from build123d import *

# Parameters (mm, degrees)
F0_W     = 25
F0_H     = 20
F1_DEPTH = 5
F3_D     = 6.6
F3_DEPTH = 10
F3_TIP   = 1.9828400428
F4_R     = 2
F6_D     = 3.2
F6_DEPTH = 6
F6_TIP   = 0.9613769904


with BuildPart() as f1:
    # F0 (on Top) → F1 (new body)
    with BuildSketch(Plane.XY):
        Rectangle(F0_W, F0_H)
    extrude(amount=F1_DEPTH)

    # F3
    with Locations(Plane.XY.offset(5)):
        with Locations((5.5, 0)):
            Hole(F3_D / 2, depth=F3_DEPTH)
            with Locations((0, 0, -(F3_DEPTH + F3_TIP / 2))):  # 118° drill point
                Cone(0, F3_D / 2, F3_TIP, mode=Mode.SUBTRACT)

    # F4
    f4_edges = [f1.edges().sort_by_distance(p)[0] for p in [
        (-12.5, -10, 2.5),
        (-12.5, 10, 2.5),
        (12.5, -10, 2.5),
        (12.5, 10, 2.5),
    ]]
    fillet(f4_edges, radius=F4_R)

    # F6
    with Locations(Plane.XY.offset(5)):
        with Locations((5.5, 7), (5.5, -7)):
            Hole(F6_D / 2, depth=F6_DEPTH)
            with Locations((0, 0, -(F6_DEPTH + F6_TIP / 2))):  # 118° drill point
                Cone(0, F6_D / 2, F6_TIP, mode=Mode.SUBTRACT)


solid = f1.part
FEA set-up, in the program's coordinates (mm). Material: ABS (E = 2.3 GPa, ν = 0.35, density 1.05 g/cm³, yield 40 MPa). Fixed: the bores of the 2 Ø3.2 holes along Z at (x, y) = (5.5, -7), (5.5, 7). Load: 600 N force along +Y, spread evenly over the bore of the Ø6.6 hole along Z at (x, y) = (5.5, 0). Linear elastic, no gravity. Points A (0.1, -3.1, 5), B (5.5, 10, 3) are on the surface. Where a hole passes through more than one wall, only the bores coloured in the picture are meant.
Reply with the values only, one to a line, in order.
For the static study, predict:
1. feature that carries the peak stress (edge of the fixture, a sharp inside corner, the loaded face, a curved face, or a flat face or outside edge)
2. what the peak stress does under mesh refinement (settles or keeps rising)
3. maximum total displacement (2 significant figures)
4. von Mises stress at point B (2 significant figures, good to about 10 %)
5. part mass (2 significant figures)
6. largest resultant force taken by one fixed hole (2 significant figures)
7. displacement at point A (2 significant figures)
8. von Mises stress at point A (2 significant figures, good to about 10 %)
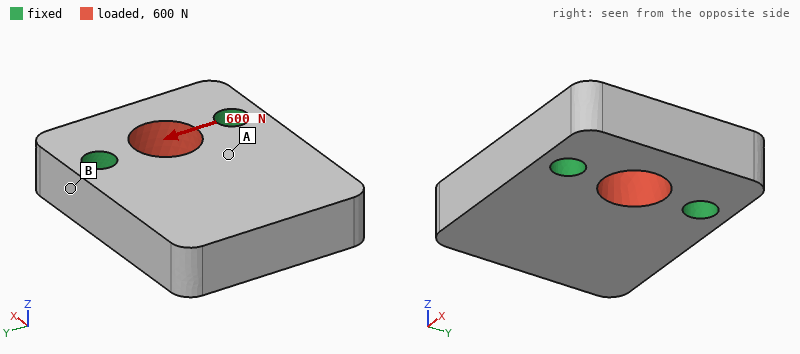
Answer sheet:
edge of the fixture
keeps rising
26 µm
4.4 MPa
2.3 g
300 N
14 µm
1.7 MPa
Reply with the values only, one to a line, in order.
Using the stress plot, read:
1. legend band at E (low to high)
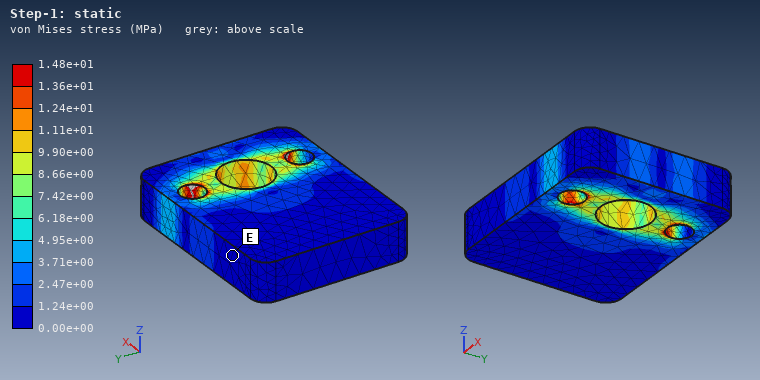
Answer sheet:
0.00e+00 to 1.24e+00 MPa
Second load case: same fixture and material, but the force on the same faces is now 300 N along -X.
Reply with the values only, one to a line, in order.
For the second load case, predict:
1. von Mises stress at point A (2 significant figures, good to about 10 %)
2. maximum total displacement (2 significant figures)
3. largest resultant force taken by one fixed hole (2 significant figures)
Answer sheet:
2.2 MPa
20 µm
150 N
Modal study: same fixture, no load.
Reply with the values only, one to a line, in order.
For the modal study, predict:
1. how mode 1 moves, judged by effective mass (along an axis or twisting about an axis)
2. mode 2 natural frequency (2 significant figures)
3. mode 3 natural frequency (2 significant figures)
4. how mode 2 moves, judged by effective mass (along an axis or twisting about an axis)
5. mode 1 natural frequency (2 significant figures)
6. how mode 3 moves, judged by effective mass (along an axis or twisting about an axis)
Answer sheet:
along Z
7300 Hz
9100 Hz
twisting about X
3400 Hz
along Y
